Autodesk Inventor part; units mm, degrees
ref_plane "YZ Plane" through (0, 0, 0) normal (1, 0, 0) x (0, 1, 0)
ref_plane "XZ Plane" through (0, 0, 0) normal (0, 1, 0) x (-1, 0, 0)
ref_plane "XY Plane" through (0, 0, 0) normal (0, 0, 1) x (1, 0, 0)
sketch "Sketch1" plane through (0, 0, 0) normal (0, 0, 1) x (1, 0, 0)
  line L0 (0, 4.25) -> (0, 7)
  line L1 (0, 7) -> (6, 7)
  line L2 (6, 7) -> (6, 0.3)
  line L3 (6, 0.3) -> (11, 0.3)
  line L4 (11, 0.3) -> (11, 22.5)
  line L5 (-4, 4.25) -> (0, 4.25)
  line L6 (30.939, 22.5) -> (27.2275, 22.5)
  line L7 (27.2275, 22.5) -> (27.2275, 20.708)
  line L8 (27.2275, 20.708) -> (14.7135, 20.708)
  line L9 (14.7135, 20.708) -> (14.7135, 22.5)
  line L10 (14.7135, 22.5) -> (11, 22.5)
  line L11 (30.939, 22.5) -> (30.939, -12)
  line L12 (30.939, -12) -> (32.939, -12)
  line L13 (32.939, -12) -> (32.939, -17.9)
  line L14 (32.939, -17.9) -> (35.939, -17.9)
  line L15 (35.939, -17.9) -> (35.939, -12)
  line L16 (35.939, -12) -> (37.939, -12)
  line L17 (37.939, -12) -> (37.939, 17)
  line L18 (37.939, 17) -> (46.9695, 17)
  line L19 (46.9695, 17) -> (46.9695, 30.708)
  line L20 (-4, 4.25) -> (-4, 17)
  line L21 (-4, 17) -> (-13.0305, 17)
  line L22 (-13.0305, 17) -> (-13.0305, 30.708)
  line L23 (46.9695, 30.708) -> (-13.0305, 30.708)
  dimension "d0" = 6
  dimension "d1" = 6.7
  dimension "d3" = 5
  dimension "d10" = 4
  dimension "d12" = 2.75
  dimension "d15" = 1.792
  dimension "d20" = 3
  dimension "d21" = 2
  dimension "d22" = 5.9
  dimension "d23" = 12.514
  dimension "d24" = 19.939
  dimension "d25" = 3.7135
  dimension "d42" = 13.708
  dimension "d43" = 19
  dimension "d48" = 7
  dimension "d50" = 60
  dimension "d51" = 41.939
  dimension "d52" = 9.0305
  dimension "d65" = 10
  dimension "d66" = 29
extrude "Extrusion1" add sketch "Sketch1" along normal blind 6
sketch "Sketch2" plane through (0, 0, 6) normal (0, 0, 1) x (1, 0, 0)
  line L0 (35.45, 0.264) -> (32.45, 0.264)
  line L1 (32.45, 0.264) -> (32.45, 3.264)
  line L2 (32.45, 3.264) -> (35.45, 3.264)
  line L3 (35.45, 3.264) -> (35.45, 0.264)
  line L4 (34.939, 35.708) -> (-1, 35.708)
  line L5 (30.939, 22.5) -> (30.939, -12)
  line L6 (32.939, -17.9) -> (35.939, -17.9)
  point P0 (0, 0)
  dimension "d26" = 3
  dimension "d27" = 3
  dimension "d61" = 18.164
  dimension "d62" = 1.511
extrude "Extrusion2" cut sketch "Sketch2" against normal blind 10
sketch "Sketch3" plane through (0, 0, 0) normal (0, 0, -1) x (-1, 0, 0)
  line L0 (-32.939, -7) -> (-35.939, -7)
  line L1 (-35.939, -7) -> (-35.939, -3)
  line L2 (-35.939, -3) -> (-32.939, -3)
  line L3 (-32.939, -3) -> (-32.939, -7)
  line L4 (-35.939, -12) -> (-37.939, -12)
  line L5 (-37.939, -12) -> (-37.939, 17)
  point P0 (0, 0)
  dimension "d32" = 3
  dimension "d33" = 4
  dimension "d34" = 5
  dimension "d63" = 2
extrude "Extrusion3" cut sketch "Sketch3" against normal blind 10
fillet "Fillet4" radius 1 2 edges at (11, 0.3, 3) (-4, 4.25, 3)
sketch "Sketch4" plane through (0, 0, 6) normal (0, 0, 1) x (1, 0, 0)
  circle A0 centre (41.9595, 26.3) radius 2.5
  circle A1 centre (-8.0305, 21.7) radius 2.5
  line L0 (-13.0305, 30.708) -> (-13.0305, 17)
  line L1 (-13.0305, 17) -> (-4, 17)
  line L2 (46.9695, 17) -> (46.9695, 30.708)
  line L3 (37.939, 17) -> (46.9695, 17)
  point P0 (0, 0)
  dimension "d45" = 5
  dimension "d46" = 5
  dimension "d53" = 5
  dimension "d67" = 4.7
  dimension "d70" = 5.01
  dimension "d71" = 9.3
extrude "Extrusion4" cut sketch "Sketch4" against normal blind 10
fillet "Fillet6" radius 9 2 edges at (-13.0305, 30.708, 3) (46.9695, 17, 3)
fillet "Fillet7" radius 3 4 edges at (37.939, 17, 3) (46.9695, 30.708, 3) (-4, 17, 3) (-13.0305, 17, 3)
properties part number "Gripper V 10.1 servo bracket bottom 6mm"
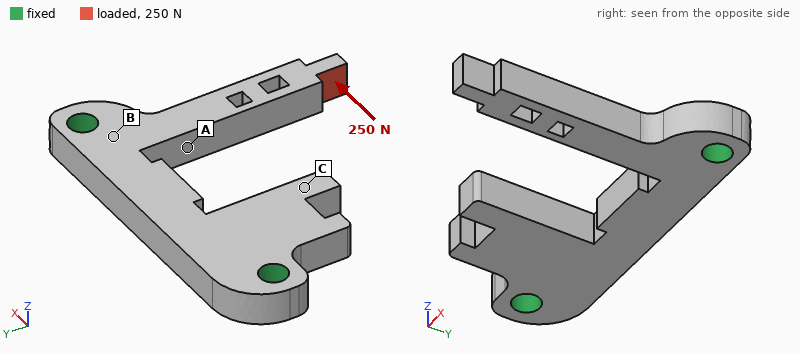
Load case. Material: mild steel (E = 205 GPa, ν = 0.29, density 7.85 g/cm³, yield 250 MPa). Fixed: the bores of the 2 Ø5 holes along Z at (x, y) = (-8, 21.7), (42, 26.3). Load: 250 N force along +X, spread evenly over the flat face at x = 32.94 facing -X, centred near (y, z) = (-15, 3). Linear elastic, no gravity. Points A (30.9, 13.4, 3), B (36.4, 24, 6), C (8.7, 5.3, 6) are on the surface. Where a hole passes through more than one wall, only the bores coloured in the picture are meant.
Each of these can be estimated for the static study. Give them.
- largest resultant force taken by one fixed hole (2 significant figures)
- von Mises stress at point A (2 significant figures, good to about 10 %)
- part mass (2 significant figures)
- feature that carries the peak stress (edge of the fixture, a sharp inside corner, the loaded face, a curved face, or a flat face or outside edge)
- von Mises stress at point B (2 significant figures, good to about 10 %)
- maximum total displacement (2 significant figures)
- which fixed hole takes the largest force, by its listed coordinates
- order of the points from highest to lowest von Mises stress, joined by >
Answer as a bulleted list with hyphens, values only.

- 380 N
- 140 MPa
- 50 g
- a curved face
- 37 MPa
- 0.14 mm
- (42, 26.3)
- A > B > C
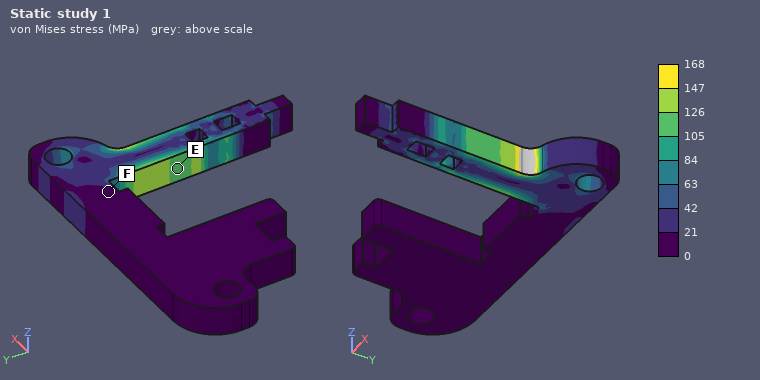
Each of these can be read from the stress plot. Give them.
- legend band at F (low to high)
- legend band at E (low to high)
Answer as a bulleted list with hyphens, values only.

- 0 to 21 MPa
- 105 to 126 MPa
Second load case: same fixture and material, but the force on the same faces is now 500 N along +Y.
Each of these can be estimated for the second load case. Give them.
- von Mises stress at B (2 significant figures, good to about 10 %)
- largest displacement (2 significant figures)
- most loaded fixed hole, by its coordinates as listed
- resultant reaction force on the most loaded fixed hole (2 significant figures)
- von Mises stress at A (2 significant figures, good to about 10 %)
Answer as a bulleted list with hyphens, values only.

- 15 MPa
- 28 µm
- (42, 26.3)
- 460 N
- 27 MPa
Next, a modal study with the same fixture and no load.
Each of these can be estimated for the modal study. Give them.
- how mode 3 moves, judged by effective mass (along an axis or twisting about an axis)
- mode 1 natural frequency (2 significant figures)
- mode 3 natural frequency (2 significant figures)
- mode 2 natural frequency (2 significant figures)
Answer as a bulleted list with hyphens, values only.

- along Z
- 3300 Hz
- 8800 Hz
- 4500 Hz
